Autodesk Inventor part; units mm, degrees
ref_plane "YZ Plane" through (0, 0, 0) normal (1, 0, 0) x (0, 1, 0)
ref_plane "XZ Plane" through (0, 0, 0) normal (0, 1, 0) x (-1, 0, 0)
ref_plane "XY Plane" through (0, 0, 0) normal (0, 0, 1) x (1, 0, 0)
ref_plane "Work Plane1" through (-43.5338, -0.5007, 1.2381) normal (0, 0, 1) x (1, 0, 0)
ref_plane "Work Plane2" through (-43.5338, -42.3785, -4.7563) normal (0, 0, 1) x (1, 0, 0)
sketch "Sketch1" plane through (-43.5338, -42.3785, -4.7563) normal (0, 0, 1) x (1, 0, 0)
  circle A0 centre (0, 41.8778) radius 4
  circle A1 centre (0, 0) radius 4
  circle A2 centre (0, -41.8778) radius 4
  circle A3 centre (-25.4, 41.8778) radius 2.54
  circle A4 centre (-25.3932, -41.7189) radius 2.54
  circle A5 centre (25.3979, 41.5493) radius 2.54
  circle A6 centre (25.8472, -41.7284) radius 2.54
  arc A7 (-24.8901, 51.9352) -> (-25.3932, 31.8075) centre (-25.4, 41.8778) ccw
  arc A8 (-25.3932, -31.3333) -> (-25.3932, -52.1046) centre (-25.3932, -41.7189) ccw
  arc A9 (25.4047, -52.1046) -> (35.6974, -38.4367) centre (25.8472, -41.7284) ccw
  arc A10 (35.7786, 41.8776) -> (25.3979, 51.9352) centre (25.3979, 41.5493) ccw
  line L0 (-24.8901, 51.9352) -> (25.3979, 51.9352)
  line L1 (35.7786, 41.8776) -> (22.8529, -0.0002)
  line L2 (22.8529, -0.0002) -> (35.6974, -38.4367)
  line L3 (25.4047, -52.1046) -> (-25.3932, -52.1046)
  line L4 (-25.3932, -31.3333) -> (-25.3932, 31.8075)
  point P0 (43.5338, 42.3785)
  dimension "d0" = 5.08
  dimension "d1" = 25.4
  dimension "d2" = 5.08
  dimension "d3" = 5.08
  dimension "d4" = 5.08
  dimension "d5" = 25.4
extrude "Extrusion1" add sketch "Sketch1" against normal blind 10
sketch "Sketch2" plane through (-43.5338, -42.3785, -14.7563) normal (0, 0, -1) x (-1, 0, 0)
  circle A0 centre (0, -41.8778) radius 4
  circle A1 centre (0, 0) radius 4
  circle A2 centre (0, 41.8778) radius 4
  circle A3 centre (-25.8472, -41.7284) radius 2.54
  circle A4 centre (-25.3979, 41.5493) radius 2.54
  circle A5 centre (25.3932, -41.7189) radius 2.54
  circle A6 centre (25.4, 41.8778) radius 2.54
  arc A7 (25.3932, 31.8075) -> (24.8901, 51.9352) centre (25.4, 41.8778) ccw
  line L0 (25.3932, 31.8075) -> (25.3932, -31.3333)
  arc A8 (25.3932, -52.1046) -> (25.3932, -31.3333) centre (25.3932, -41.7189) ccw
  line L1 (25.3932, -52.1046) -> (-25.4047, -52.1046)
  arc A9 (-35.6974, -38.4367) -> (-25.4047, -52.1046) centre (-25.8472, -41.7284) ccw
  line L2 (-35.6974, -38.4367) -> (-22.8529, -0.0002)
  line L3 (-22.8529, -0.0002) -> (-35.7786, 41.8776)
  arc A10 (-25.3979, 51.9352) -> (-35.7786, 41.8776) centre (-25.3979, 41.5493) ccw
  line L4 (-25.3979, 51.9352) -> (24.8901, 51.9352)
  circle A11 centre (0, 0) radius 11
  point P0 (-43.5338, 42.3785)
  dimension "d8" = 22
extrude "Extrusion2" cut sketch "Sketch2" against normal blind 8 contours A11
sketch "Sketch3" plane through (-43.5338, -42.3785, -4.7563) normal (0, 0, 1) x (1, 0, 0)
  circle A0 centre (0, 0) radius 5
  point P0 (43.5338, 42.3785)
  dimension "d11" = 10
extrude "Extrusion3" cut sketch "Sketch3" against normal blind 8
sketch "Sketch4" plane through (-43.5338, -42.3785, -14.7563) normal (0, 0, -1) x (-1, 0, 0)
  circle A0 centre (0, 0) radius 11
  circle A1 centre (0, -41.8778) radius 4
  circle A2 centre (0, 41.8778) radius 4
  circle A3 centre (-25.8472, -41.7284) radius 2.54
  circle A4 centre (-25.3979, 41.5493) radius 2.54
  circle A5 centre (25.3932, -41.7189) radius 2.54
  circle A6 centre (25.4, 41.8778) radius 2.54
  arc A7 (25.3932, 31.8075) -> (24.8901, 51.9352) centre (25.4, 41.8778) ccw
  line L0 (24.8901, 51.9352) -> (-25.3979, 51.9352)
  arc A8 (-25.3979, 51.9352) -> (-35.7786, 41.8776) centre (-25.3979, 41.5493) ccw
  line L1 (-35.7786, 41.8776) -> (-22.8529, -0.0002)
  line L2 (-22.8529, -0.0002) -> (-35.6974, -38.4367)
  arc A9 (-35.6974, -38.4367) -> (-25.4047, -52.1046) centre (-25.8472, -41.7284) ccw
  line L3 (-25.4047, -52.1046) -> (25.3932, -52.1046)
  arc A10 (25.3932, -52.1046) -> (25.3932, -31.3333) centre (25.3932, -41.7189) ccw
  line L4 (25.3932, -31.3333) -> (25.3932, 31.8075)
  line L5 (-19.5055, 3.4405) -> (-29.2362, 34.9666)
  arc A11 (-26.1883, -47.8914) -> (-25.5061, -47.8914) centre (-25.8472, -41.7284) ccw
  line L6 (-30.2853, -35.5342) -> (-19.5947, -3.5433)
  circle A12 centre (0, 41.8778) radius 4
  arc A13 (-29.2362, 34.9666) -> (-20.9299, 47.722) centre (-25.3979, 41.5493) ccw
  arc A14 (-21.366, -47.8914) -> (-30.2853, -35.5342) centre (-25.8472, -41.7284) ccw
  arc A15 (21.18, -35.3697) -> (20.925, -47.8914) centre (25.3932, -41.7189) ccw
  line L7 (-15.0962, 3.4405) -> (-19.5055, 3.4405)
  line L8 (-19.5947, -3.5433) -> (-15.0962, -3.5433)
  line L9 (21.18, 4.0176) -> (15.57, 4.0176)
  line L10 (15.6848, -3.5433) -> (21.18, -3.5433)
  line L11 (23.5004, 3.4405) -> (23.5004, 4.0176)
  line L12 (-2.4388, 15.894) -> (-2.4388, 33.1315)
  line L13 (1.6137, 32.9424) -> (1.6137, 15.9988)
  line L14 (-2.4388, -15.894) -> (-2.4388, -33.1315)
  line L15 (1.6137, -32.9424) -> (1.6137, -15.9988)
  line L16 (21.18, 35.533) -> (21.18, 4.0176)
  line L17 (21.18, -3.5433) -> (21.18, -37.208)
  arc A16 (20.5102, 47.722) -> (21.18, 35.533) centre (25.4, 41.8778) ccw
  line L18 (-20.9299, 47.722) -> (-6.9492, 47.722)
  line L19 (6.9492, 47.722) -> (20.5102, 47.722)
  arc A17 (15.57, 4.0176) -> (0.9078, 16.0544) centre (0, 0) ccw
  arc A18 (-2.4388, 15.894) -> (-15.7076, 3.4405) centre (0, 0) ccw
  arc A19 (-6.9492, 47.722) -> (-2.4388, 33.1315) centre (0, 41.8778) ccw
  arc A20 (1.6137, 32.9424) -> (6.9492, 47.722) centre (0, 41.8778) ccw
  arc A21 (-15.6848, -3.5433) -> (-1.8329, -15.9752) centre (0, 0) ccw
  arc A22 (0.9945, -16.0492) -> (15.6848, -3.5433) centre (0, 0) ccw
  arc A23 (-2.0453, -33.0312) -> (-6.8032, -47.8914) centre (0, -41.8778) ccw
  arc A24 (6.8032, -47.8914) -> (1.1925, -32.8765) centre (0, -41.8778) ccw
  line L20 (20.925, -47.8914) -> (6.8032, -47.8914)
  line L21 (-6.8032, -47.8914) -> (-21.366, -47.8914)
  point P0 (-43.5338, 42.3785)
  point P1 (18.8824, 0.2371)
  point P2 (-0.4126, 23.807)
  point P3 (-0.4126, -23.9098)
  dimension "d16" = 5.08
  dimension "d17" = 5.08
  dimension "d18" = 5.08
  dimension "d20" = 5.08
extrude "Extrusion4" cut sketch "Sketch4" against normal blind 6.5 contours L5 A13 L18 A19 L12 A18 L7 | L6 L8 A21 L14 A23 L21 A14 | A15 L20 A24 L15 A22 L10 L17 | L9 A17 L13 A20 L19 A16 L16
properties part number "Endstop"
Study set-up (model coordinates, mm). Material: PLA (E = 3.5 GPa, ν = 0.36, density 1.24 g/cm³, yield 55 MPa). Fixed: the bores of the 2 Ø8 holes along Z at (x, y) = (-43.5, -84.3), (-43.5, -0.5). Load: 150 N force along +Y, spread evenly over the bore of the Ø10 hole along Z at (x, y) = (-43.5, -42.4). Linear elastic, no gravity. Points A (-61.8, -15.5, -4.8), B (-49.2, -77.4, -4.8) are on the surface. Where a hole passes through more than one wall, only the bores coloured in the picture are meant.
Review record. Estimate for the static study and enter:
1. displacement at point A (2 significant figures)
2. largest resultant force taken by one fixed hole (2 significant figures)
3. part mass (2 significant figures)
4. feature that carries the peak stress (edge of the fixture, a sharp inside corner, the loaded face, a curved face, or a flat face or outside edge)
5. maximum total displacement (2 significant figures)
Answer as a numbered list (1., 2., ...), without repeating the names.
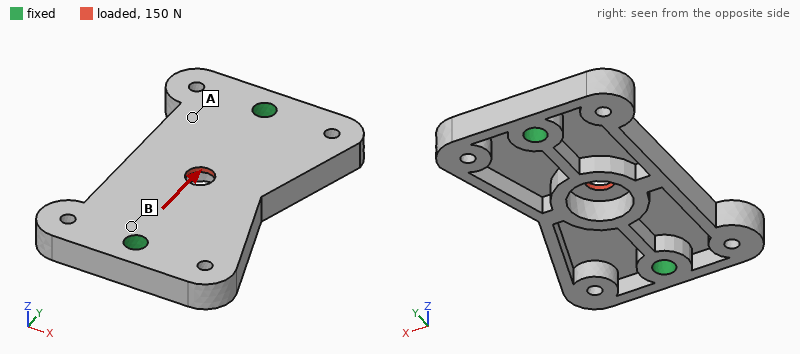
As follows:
1. 3.4 µm
2. 75 N
3. 48 g
4. the loaded face
5. 11 µm
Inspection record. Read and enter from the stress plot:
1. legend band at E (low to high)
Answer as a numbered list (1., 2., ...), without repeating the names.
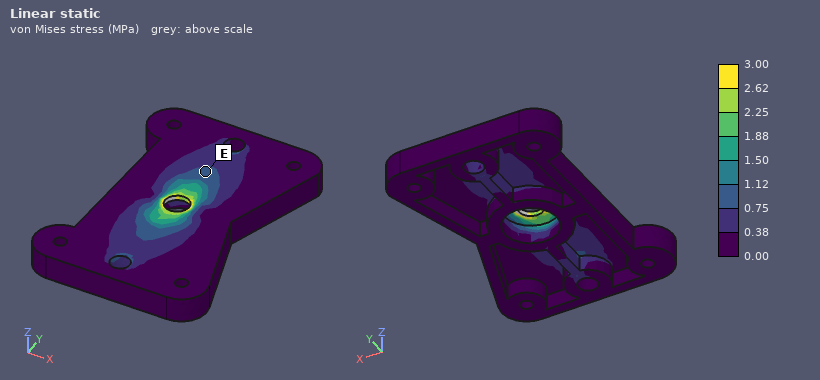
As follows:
1. 0.75 to 1.12 MPa
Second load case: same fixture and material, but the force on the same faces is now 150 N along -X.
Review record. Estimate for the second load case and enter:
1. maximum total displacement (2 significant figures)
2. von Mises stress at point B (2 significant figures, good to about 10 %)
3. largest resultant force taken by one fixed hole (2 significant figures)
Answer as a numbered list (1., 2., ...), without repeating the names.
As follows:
1. 24 µm
2. 1.00 MPa
3. 75 N
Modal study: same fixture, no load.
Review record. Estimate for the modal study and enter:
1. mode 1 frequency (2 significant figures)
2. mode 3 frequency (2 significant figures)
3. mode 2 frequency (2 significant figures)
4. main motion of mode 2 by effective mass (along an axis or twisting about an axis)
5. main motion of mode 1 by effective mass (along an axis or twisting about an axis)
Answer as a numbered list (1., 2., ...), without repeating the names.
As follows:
1. 1100 Hz
2. 1700 Hz
3. 1300 Hz
4. along Z
5. twisting about Y
